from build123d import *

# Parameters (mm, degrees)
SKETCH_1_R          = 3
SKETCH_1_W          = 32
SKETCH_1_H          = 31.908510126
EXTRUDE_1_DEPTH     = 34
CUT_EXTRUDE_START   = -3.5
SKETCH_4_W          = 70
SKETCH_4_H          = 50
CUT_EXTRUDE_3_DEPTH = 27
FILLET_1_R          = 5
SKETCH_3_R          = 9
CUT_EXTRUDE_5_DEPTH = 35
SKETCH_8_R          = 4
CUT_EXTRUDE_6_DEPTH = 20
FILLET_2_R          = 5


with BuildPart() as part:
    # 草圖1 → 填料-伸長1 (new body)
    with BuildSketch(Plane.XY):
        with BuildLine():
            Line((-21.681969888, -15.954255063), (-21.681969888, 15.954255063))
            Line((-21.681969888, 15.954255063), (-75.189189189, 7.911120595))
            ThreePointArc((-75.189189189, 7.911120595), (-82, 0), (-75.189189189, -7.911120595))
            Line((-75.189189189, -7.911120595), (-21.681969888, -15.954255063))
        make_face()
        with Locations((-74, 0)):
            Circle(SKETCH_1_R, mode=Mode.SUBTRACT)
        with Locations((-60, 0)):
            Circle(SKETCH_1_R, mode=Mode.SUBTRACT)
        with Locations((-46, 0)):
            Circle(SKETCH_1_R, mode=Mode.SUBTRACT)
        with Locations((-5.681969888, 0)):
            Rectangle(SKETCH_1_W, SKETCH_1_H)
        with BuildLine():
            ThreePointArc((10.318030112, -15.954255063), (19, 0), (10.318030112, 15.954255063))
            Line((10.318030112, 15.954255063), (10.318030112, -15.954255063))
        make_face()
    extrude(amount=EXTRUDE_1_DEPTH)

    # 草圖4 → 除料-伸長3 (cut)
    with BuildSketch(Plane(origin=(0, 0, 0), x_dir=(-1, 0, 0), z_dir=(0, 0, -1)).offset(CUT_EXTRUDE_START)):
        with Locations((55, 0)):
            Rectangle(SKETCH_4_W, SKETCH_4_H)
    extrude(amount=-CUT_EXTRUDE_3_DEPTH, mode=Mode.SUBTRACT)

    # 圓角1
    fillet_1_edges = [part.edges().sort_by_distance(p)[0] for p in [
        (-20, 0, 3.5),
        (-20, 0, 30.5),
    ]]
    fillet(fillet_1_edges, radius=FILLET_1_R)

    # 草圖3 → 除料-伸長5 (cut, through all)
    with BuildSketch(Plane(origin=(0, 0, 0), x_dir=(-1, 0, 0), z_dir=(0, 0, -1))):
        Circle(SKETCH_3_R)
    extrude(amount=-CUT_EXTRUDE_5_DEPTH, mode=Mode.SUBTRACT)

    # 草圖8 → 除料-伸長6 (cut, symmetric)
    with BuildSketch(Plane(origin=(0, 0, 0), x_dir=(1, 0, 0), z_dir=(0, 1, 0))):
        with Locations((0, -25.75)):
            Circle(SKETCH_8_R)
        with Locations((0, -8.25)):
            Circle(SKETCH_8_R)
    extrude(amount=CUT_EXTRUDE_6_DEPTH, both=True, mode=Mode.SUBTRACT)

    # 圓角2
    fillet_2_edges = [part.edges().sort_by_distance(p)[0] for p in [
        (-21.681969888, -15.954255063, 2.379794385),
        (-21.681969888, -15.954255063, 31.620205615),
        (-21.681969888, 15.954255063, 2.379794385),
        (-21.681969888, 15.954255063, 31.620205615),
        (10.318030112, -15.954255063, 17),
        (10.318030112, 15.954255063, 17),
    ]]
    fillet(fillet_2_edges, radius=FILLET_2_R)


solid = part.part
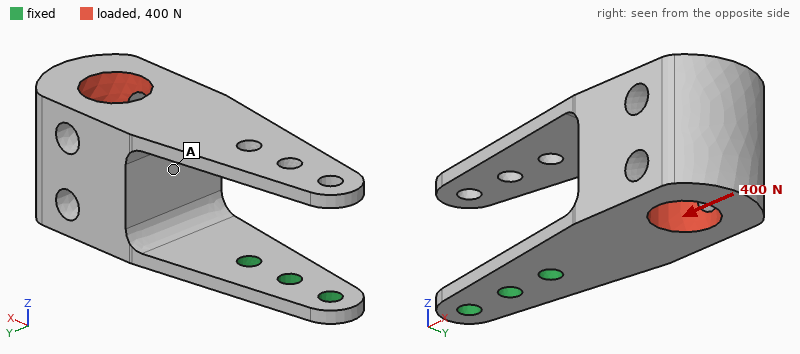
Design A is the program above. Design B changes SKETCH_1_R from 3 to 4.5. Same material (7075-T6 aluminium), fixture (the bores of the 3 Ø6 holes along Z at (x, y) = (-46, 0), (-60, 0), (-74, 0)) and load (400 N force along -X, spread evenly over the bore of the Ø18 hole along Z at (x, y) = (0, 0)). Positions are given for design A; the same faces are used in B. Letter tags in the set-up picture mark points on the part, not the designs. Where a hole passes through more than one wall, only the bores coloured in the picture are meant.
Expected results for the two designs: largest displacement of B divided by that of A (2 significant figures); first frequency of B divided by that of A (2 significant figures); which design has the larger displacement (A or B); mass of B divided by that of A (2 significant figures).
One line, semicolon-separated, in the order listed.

0.90; 1.1; A; 0.98
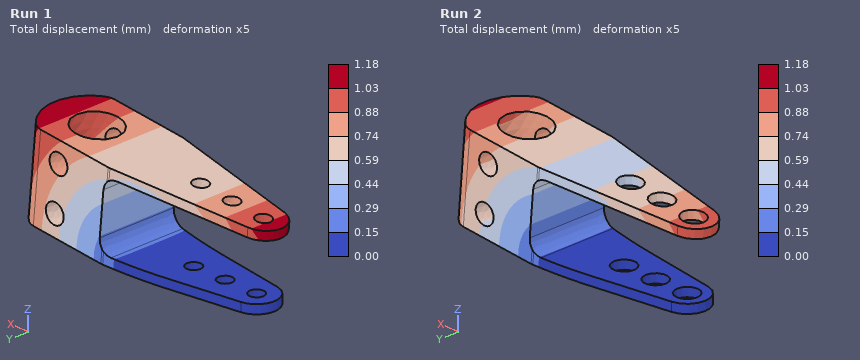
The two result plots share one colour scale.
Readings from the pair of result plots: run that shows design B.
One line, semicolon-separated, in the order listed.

Run 2
